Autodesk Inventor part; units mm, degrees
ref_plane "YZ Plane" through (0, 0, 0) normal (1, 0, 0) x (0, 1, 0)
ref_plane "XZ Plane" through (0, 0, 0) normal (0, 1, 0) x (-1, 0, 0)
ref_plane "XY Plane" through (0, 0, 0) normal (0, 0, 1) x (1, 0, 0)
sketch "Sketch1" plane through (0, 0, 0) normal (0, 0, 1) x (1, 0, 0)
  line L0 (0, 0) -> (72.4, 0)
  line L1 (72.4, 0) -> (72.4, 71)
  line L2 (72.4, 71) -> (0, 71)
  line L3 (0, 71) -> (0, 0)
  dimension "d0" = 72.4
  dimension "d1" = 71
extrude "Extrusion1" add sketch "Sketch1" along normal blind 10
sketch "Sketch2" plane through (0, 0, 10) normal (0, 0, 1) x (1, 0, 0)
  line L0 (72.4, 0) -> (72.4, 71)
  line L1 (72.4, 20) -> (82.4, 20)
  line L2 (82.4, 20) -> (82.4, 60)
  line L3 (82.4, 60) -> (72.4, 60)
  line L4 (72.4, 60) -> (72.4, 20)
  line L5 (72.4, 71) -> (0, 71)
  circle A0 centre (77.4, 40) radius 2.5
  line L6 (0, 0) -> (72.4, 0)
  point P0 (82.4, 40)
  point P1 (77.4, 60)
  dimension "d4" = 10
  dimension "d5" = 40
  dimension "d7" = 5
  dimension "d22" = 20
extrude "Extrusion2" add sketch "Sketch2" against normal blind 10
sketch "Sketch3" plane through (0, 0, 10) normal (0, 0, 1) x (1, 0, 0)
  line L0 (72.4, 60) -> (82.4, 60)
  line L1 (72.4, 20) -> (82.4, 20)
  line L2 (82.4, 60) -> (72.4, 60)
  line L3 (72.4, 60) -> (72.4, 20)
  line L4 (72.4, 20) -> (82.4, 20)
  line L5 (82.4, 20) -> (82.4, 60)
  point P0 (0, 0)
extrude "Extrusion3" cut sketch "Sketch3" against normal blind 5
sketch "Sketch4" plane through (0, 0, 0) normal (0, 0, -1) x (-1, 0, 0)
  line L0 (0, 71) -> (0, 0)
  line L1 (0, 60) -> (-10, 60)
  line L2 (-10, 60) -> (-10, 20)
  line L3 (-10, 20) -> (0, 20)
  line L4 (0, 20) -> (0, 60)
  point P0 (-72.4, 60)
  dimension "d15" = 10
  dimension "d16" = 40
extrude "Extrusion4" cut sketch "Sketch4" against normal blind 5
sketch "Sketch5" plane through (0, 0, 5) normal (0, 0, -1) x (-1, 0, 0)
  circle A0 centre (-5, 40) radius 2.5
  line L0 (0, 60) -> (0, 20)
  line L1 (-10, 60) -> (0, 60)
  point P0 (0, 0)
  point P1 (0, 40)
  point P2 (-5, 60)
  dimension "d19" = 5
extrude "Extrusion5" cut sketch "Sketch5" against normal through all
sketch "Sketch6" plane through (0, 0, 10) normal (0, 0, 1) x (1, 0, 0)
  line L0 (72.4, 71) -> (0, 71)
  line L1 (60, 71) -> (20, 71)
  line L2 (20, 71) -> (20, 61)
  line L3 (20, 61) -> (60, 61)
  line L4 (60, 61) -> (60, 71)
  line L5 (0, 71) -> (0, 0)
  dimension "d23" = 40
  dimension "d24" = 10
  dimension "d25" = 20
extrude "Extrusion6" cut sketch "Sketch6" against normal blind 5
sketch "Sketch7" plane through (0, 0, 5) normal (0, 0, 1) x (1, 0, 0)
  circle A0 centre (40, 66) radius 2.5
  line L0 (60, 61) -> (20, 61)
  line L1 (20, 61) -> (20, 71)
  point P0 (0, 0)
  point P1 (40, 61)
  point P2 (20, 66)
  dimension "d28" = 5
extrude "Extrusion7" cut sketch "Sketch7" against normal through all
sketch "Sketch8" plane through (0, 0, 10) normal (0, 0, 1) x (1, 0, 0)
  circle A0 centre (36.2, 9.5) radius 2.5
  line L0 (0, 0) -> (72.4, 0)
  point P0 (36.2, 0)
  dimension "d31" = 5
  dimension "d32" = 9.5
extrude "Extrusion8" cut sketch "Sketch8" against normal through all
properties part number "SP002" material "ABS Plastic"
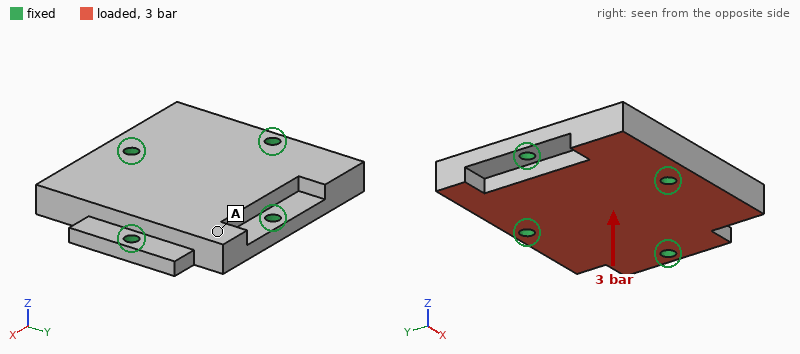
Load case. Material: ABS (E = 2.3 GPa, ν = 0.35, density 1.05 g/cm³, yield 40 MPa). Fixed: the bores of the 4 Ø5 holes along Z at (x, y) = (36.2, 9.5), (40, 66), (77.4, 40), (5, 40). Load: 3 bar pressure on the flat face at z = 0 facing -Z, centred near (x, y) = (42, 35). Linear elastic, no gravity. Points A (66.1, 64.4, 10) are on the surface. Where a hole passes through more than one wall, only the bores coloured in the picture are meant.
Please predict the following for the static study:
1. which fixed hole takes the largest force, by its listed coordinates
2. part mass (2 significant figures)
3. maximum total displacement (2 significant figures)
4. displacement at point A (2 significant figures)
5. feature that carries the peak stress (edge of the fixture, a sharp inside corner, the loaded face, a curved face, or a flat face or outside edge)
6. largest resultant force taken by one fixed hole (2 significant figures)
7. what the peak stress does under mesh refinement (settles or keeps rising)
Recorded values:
(36.2, 9.5)
51 g
0.20 mm
0.11 mm
edge of the fixture
550 N
keeps rising
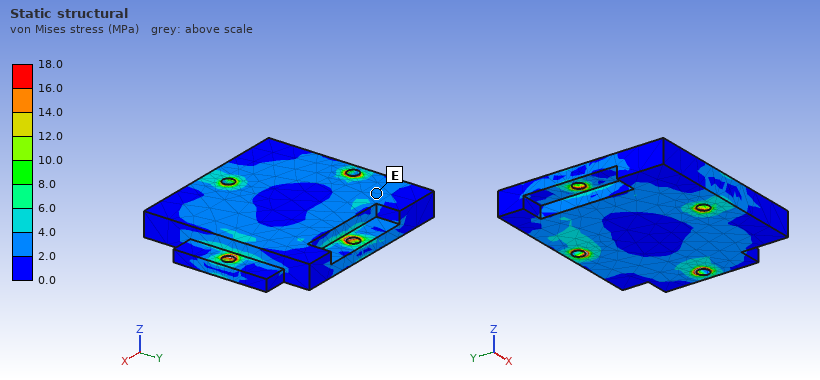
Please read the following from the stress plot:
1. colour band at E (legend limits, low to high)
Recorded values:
2.0 to 4.0 MPa
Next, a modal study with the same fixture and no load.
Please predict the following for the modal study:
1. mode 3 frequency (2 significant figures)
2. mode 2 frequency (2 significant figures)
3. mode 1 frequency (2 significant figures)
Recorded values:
2600 Hz
2400 Hz
2200 Hz
